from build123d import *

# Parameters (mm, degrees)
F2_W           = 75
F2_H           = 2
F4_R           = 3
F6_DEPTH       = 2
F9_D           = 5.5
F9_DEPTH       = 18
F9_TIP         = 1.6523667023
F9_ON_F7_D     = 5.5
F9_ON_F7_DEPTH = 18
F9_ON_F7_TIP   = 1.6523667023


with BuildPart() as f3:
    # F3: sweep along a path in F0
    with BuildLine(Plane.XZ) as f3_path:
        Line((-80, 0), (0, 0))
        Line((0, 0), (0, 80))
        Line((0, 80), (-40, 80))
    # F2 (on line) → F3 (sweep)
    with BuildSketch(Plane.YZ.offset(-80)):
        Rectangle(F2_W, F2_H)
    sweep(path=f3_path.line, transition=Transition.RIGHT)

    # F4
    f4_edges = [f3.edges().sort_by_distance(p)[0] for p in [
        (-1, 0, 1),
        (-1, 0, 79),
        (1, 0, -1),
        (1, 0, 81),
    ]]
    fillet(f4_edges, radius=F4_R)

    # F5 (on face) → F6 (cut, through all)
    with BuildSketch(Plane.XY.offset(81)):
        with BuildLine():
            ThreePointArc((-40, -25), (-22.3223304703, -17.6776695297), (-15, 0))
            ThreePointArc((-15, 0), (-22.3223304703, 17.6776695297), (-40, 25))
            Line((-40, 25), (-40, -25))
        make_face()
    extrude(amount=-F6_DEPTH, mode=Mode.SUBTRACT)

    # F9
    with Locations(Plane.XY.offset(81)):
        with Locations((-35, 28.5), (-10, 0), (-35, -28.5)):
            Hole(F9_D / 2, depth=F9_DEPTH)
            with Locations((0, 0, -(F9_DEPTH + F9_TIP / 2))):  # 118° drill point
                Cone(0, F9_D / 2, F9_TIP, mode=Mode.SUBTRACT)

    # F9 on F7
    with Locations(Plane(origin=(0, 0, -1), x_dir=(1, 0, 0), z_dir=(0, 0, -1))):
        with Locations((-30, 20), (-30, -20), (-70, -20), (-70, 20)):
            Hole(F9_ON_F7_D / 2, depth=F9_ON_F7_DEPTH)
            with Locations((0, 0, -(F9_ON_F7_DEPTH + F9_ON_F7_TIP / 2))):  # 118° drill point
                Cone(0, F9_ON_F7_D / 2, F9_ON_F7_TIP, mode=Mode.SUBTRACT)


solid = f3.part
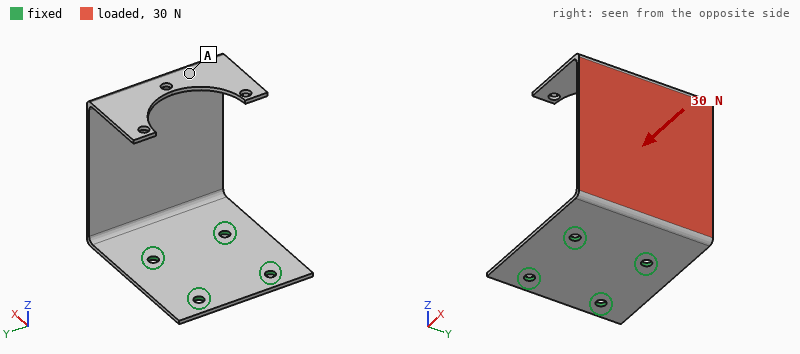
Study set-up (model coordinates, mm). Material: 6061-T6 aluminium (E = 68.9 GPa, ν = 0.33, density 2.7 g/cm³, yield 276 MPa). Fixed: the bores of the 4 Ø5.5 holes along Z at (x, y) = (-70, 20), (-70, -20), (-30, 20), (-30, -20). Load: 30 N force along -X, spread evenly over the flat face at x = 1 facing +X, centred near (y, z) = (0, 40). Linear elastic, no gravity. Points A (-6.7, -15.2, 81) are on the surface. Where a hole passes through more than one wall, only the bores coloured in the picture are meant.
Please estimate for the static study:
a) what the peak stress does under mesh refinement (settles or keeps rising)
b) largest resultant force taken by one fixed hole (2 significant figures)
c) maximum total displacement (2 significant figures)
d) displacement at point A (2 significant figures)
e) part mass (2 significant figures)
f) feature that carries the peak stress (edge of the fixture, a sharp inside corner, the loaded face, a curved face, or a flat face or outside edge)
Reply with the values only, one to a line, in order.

keeps rising
13 N
1.3 mm
1.2 mm
75 g
edge of the fixture
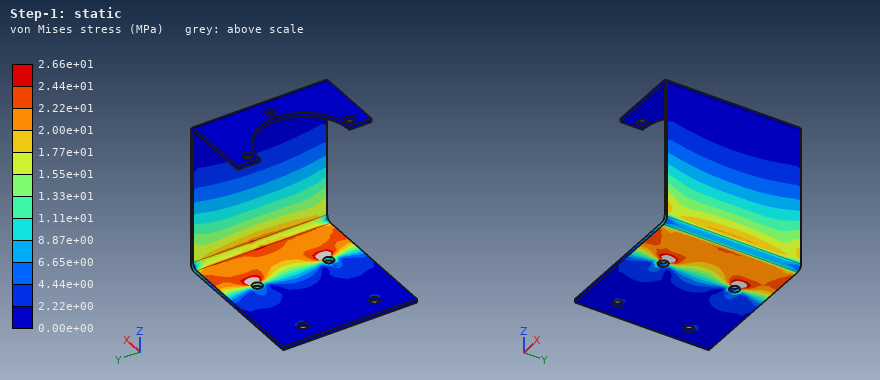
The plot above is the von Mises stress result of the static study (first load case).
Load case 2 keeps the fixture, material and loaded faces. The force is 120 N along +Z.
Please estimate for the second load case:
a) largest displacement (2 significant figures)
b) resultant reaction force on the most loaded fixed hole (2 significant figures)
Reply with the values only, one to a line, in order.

1.4 mm
69 N
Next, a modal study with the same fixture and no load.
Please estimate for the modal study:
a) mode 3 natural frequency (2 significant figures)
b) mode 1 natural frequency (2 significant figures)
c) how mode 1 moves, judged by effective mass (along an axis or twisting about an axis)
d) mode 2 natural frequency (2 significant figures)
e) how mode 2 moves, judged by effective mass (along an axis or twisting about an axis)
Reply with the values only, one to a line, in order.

460 Hz
120 Hz
along X
260 Hz
along Y
